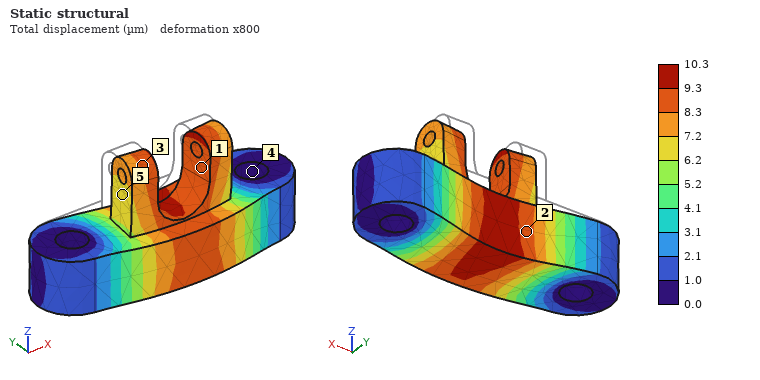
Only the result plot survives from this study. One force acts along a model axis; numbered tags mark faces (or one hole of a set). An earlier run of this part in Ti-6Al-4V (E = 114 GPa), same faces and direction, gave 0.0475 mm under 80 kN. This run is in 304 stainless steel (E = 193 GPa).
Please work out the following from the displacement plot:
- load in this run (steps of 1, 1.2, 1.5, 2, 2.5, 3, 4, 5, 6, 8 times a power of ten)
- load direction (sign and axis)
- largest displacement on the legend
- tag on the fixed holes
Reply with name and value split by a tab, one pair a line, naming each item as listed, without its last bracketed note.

load in this run	30 kN
load direction	-Y
largest displacement on the legend	10.3 µm
tag on the fixed holes	4
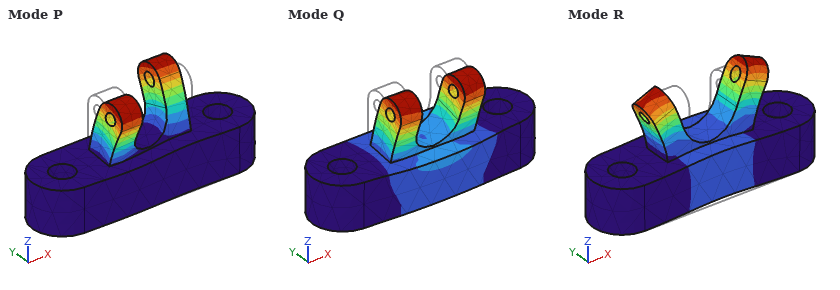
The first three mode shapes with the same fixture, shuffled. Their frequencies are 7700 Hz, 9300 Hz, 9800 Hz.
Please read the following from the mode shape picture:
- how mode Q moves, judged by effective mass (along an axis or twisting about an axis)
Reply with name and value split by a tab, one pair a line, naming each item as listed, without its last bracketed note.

how mode Q moves, judged by effective mass	along Y
